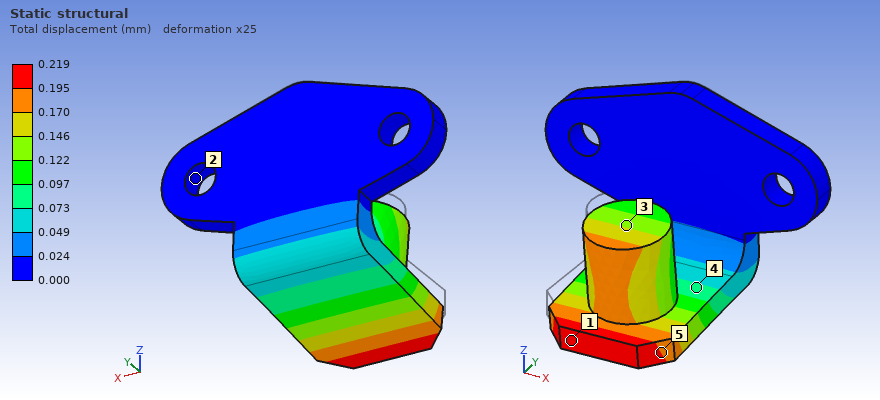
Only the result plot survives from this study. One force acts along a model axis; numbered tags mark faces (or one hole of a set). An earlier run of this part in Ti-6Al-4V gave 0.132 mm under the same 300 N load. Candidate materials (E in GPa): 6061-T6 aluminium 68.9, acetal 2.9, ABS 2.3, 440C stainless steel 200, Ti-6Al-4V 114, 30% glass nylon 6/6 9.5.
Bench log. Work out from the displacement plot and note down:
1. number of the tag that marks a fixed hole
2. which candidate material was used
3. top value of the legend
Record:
2
6061-T6 aluminium
0.219 mm
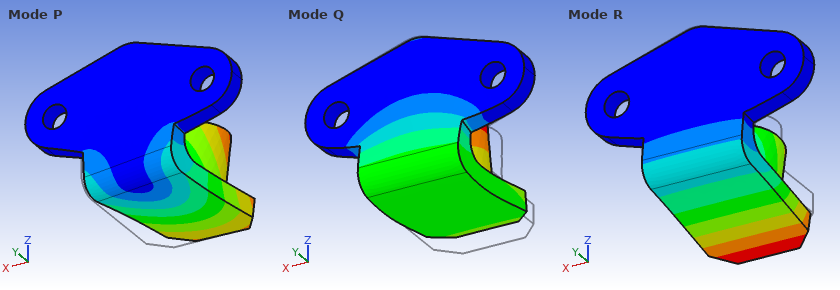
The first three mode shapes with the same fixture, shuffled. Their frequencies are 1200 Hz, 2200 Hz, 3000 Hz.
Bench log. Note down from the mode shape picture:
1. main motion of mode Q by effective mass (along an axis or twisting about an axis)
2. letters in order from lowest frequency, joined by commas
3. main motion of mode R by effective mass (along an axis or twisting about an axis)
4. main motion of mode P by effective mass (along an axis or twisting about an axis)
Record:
along Y
R, P, Q
along Z
along X
